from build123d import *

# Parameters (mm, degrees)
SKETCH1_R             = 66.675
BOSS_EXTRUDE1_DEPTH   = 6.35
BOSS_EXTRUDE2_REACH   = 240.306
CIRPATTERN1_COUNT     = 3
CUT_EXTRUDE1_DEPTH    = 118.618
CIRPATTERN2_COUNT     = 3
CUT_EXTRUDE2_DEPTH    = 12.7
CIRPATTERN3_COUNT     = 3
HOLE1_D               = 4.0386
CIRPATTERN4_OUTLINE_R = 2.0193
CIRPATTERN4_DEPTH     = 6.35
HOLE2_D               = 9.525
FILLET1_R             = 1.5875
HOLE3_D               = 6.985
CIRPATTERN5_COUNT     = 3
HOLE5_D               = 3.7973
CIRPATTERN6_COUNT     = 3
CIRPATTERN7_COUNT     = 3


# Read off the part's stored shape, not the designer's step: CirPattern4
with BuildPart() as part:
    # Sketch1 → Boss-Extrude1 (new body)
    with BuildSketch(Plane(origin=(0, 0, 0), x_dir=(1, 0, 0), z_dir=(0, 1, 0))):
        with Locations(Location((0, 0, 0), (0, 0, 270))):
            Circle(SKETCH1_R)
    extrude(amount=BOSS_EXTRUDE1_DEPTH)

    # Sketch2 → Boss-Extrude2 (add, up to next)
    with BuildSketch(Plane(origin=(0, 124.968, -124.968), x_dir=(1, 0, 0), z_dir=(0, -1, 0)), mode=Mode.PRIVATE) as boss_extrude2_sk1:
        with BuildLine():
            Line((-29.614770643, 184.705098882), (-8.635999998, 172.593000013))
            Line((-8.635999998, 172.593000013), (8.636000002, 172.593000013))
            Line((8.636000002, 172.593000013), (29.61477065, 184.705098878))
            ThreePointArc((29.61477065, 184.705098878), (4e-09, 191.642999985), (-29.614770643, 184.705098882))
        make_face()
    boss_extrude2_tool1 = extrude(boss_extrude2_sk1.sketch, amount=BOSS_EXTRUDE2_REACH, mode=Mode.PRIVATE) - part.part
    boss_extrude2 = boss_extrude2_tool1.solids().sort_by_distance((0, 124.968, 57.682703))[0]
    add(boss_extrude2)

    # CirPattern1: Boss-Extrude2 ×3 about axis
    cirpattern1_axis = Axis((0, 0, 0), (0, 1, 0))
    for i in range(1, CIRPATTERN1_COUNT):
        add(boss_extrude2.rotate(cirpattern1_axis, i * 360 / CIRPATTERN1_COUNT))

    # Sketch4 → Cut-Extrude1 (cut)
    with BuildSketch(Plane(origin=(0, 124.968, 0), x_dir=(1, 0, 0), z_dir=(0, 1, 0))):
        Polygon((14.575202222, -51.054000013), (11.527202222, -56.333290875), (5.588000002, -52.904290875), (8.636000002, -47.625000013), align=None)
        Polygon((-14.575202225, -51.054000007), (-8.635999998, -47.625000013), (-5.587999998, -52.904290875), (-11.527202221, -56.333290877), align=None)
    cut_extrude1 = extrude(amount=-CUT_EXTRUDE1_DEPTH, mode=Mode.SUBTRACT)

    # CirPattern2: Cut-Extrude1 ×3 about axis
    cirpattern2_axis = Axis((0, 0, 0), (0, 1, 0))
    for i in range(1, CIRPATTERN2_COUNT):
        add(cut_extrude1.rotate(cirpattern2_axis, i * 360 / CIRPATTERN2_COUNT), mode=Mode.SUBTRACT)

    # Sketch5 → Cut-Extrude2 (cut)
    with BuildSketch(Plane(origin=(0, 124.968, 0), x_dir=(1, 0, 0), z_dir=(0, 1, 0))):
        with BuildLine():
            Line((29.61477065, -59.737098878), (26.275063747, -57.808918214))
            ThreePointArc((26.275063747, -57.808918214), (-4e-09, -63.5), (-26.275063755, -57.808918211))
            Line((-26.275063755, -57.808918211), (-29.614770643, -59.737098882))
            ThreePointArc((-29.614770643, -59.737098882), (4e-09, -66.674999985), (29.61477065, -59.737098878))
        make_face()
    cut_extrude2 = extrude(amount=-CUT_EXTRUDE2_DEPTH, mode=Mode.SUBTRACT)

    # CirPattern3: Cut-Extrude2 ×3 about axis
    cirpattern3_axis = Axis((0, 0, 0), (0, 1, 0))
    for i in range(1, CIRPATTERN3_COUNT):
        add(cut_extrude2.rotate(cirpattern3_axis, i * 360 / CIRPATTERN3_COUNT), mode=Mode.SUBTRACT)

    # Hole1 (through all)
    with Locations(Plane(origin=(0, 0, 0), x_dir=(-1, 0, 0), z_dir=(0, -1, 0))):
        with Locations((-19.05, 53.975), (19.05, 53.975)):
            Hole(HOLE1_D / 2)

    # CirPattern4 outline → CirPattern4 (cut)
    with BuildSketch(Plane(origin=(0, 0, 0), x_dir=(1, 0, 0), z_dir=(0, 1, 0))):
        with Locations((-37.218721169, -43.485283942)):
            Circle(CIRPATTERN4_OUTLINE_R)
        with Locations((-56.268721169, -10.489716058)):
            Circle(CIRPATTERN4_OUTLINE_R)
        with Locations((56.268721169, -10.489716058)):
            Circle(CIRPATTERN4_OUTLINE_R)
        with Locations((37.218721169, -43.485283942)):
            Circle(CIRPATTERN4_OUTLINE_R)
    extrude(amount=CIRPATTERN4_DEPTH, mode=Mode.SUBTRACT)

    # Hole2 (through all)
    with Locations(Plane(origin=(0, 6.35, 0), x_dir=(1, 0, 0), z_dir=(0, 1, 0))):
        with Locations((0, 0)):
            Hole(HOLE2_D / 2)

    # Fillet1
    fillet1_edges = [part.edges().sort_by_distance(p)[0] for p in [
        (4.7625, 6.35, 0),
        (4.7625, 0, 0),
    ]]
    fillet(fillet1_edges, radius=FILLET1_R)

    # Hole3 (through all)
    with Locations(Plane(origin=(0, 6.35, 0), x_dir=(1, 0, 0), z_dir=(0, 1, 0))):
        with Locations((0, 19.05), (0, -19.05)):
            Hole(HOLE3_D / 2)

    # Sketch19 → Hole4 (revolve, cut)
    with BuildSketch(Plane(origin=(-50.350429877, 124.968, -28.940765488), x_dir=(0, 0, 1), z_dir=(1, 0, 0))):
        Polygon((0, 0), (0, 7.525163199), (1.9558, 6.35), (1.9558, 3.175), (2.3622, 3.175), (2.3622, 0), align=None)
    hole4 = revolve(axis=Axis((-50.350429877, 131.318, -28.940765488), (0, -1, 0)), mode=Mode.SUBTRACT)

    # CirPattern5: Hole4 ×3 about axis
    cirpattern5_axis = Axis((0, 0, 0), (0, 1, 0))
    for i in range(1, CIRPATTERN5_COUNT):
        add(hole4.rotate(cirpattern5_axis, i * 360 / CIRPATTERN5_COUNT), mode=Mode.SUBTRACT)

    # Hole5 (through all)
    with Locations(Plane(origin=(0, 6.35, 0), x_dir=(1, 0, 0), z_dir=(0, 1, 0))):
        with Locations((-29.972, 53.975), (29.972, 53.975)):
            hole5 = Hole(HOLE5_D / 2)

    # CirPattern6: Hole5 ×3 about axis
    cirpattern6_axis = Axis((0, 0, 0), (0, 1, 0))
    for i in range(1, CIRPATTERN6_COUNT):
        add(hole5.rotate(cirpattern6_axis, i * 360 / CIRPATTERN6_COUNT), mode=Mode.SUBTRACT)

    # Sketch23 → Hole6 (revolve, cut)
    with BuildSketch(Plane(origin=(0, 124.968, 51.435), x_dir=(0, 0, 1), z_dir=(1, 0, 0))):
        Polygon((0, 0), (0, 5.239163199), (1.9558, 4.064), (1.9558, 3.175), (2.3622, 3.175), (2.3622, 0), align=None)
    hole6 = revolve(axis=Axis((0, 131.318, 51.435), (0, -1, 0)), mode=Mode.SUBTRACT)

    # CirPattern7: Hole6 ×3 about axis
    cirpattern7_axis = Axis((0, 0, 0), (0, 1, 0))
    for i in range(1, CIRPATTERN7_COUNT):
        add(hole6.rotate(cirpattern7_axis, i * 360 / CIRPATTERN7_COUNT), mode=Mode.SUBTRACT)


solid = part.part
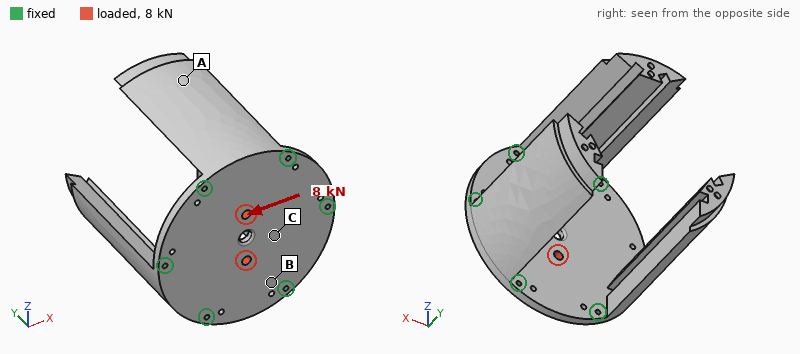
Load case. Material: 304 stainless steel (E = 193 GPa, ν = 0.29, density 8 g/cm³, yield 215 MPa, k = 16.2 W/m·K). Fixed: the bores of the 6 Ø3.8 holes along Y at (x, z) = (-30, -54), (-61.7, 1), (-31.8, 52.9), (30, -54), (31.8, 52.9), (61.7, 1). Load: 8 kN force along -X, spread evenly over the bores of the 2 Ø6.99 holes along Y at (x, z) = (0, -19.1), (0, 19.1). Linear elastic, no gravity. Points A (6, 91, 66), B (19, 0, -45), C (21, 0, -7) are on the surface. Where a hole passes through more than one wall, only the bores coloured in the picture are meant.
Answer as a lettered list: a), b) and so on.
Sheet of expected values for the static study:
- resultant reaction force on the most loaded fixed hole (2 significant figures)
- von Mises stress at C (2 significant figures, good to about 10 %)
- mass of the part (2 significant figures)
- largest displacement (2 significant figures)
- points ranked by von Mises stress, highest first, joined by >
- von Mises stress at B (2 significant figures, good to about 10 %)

a) 1.7 kN
b) 6.4 MPa
c) 2.5 kg
d) 3.9 µm
e) B > C > A
f) 9.1 MPa
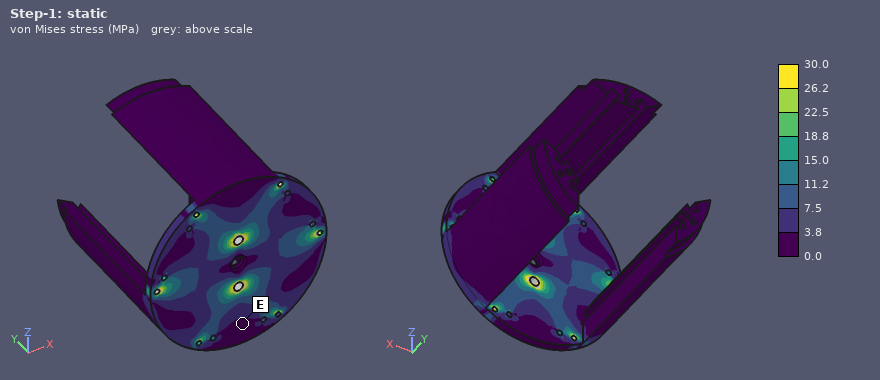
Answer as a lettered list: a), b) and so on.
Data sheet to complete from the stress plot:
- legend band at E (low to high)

a) 0.0 to 3.8 MPa
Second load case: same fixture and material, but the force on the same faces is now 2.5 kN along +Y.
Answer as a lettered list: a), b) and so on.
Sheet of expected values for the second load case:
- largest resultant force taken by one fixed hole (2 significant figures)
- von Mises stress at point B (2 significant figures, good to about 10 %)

a) 480 N
b) 17 MPa
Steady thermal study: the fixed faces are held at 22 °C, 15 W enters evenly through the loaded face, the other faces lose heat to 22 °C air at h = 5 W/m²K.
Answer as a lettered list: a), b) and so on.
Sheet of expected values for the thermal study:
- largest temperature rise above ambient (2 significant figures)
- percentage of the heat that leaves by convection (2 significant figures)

a) 45 K
b) 23 %
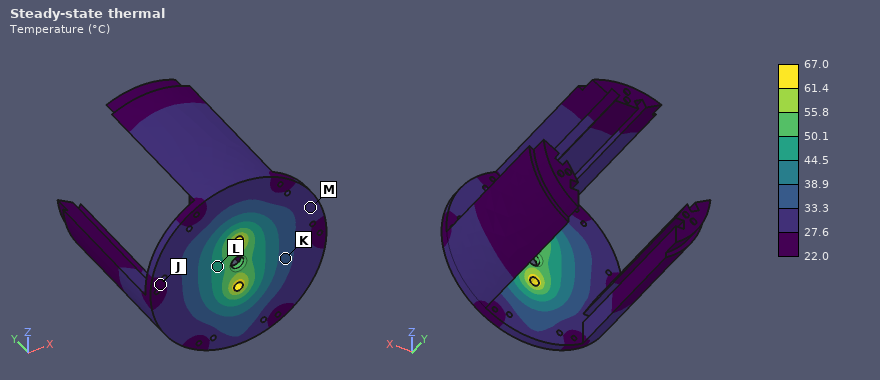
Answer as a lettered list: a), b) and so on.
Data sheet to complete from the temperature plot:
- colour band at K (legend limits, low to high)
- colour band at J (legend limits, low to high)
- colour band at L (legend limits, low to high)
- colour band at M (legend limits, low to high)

a) 33.3 to 38.9 °C
b) 22.0 to 27.6 °C
c) 44.5 to 50.1 °C
d) 27.6 to 33.3 °C
